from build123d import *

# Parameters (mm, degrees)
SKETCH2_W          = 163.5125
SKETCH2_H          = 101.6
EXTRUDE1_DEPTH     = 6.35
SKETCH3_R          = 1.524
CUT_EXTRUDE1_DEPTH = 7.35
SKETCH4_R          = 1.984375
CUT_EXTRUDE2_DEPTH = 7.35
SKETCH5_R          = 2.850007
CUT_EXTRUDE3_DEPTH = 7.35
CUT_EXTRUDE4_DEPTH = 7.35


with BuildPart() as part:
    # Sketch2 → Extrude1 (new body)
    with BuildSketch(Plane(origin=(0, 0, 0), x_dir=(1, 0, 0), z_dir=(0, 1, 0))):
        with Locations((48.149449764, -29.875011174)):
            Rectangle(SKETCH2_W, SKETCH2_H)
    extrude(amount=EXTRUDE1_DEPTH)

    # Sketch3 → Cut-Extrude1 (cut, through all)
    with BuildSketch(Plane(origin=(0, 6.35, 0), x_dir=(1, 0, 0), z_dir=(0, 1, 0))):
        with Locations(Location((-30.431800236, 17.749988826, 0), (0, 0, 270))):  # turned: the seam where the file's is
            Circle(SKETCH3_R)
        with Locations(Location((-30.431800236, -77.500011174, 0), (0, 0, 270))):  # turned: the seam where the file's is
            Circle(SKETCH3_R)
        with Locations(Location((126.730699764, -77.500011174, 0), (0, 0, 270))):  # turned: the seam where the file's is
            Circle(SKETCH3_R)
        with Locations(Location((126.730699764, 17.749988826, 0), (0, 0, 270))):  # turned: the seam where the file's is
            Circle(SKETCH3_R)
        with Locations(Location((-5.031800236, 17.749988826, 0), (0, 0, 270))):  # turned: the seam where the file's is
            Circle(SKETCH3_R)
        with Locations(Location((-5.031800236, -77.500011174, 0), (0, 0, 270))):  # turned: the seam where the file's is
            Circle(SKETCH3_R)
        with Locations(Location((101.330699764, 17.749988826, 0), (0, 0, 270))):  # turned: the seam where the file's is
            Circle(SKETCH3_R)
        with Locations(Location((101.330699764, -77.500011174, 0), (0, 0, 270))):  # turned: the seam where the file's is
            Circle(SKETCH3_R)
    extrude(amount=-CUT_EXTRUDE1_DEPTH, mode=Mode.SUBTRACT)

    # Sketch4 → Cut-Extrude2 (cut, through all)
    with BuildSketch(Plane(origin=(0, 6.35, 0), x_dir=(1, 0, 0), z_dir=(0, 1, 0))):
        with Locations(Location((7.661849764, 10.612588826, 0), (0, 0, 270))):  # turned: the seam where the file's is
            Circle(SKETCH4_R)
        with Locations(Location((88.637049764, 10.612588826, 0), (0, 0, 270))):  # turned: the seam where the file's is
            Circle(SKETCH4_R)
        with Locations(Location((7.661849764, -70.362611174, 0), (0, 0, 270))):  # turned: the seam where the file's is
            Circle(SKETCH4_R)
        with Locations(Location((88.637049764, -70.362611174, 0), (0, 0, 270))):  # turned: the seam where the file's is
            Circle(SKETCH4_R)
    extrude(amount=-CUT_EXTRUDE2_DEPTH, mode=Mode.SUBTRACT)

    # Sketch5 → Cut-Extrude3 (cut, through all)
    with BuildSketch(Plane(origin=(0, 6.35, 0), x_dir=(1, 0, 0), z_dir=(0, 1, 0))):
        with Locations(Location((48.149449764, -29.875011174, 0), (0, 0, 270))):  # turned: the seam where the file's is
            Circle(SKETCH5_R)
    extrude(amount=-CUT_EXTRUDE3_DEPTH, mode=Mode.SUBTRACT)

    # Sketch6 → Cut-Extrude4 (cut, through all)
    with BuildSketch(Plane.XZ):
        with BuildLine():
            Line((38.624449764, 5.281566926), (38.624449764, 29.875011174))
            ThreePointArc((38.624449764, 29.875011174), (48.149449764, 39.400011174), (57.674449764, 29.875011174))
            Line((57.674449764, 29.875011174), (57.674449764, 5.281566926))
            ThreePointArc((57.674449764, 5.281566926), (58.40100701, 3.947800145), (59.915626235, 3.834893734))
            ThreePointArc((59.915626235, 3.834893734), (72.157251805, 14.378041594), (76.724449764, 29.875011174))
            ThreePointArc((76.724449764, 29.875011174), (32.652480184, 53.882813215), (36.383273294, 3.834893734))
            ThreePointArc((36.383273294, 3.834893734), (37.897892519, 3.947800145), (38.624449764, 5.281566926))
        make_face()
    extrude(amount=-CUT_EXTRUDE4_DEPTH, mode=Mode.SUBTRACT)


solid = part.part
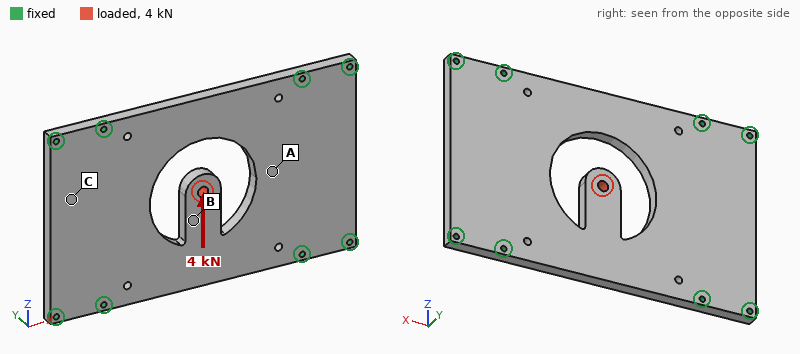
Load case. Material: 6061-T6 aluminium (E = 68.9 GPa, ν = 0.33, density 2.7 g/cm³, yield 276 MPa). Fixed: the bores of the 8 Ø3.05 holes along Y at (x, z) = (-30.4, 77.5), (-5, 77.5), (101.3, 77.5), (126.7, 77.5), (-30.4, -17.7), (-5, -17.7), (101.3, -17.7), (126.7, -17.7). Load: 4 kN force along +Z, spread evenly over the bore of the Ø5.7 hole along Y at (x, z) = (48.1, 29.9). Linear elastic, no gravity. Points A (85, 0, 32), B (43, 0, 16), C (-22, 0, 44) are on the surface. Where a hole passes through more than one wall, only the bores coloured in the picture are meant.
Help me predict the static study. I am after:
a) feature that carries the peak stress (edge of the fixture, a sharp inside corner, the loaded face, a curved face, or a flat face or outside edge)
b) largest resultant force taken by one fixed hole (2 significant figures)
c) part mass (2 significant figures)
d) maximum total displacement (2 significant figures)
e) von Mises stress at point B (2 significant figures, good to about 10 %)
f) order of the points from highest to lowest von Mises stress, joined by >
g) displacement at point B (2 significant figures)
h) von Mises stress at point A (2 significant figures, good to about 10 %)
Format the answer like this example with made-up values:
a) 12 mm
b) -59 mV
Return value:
a) a curved face
b) 1.2 kN
c) 250 g
d) 48 µm
e) 33 MPa
f) B > A > C
g) 37 µm
h) 12 MPa
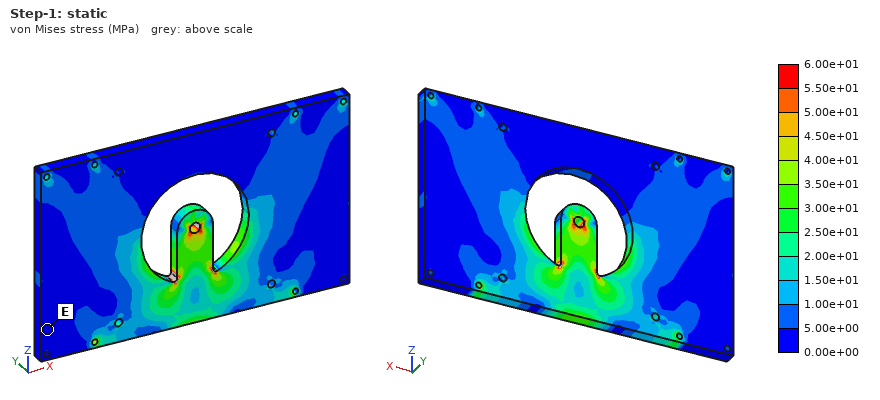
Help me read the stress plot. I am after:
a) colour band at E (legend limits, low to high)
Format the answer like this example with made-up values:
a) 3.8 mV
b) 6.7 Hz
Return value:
a) 0.00e+00 to 5.00e+00 MPa
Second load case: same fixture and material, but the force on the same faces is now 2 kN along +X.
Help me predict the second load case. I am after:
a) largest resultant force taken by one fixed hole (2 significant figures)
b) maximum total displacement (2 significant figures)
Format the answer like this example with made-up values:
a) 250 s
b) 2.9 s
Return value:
a) 1.1 kN
b) 0.17 mm
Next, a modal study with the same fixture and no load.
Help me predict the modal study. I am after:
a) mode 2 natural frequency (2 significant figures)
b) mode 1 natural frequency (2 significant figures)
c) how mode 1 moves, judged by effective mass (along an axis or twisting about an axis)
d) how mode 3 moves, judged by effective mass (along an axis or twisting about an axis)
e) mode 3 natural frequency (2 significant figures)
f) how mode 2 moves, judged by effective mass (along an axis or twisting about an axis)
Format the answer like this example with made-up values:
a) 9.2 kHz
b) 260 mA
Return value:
a) 2700 Hz
b) 1700 Hz
c) along Y
d) twisting about Z
e) 3200 Hz
f) along Y
